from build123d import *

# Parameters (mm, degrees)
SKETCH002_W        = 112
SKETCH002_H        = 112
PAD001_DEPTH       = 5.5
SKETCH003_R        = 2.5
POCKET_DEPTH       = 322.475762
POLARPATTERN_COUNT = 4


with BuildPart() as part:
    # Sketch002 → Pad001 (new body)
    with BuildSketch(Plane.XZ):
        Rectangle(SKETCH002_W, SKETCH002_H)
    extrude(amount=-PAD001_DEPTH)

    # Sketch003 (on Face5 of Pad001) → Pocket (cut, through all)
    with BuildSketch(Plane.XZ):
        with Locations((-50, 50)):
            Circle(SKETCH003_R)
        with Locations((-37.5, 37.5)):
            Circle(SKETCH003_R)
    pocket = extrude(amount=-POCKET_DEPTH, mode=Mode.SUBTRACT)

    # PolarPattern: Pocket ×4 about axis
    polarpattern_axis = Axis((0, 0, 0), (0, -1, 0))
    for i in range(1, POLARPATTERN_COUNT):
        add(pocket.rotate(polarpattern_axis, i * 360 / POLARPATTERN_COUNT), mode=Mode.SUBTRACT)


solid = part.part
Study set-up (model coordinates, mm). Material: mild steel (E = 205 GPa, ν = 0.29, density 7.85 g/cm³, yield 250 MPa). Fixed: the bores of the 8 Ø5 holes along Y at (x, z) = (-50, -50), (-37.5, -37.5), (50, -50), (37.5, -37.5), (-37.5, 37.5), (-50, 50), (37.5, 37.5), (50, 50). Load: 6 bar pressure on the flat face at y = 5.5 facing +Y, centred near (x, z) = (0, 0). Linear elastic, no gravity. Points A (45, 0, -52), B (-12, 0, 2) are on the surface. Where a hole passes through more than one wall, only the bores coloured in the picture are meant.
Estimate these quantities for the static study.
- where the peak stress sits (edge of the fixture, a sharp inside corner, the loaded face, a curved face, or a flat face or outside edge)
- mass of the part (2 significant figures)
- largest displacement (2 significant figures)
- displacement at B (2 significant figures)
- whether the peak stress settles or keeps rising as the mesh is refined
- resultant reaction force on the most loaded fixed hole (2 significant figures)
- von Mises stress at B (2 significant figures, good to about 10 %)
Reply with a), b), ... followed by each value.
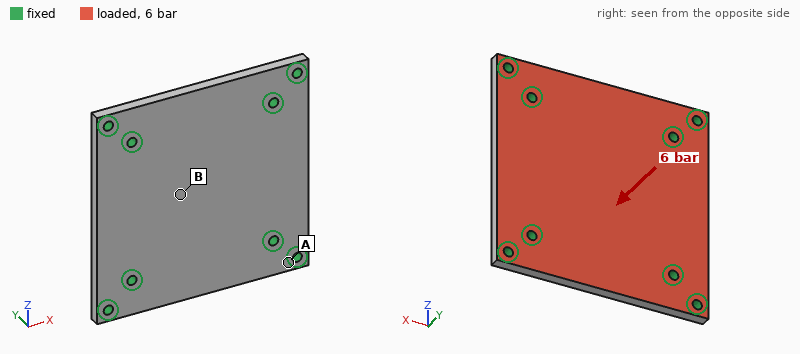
a) edge of the fixture
b) 530 g
c) 42 µm
d) 40 µm
e) keeps rising
f) 2.0 kN
g) 29 MPa
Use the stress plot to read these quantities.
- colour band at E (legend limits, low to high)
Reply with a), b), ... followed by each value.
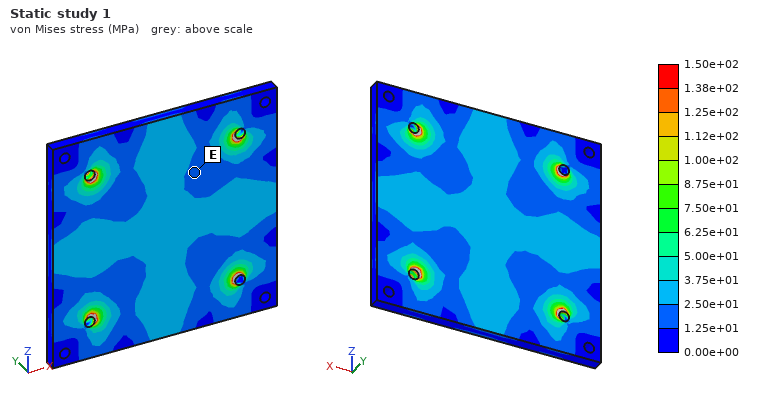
a) 1.25e+01 to 2.50e+01 MPa
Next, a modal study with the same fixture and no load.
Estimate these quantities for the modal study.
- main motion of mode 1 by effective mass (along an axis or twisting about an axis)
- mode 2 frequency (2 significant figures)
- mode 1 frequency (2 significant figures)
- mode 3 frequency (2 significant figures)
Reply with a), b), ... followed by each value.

a) along Y
b) 4800 Hz
c) 3500 Hz
d) 4900 Hz
